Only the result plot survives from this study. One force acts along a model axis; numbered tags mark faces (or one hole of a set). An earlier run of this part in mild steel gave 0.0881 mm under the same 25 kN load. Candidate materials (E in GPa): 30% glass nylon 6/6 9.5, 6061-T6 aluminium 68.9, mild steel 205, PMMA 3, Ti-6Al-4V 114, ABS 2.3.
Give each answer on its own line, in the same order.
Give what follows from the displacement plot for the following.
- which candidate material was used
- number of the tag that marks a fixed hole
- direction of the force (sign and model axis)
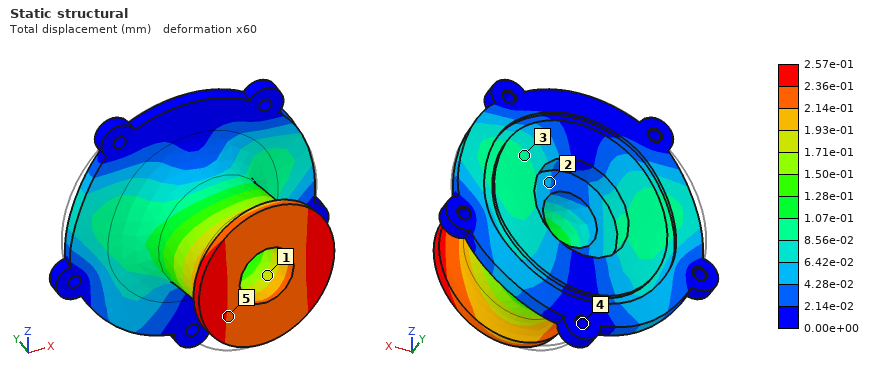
6061-T6 aluminium
4
+X
